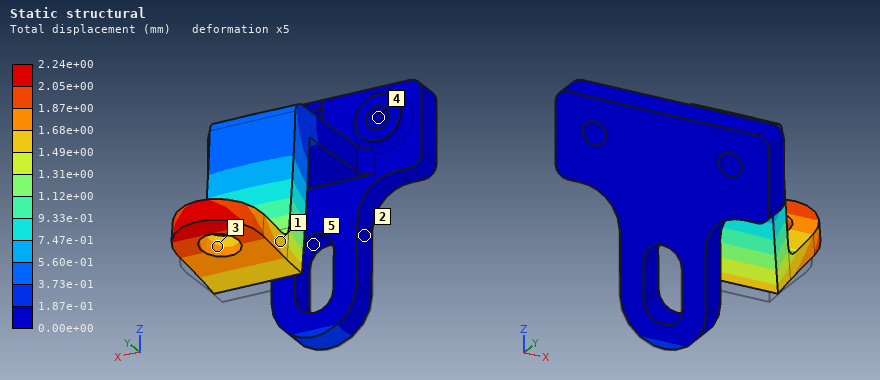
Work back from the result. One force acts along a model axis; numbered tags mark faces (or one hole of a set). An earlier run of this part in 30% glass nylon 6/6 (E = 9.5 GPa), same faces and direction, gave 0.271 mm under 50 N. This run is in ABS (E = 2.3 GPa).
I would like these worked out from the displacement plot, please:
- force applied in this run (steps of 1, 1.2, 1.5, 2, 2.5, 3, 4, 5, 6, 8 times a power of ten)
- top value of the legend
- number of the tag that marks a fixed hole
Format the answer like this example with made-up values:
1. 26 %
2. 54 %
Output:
1. 100 N
2. 2.24e+00 mm
3. 4
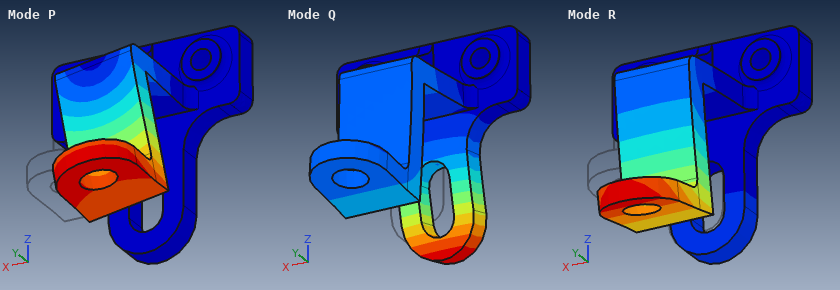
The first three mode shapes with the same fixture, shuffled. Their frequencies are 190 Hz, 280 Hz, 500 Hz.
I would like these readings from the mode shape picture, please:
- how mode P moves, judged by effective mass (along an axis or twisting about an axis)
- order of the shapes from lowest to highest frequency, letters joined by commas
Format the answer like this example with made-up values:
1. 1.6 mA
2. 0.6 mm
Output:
1. along X
2. R, P, Q
